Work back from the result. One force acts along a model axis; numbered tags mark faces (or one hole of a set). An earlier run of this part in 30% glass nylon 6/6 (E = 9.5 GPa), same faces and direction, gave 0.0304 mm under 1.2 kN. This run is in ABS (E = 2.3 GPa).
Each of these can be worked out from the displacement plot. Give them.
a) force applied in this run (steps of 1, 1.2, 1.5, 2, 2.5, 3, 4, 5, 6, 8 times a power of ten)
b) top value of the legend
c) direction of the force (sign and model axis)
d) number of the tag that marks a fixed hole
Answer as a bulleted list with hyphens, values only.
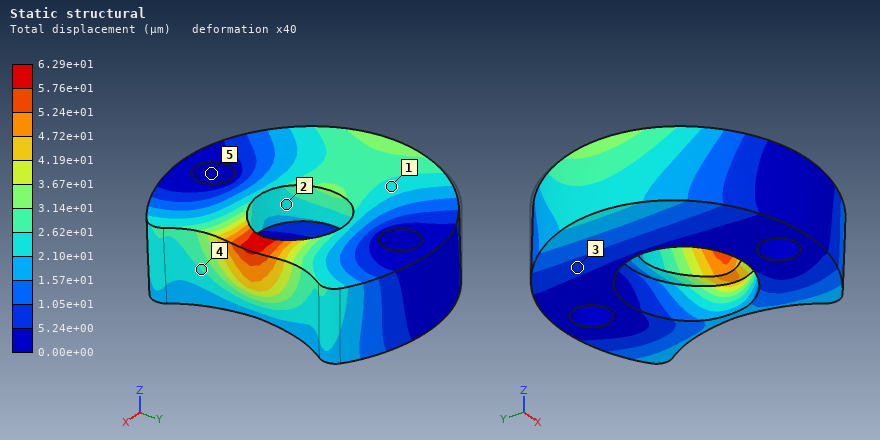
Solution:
- 600 N
- 6.29e+01 µm
- +X
- 5
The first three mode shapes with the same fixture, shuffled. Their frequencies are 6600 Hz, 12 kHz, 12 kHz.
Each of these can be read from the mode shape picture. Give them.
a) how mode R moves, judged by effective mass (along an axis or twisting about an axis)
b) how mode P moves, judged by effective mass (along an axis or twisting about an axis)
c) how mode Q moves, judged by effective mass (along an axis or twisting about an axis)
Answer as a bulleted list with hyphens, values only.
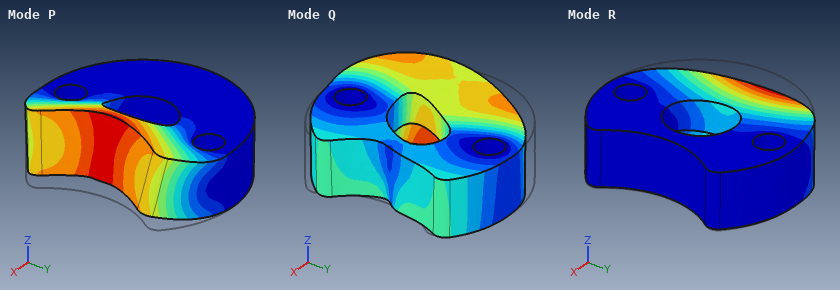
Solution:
- along Z
- along Z
- along Y
